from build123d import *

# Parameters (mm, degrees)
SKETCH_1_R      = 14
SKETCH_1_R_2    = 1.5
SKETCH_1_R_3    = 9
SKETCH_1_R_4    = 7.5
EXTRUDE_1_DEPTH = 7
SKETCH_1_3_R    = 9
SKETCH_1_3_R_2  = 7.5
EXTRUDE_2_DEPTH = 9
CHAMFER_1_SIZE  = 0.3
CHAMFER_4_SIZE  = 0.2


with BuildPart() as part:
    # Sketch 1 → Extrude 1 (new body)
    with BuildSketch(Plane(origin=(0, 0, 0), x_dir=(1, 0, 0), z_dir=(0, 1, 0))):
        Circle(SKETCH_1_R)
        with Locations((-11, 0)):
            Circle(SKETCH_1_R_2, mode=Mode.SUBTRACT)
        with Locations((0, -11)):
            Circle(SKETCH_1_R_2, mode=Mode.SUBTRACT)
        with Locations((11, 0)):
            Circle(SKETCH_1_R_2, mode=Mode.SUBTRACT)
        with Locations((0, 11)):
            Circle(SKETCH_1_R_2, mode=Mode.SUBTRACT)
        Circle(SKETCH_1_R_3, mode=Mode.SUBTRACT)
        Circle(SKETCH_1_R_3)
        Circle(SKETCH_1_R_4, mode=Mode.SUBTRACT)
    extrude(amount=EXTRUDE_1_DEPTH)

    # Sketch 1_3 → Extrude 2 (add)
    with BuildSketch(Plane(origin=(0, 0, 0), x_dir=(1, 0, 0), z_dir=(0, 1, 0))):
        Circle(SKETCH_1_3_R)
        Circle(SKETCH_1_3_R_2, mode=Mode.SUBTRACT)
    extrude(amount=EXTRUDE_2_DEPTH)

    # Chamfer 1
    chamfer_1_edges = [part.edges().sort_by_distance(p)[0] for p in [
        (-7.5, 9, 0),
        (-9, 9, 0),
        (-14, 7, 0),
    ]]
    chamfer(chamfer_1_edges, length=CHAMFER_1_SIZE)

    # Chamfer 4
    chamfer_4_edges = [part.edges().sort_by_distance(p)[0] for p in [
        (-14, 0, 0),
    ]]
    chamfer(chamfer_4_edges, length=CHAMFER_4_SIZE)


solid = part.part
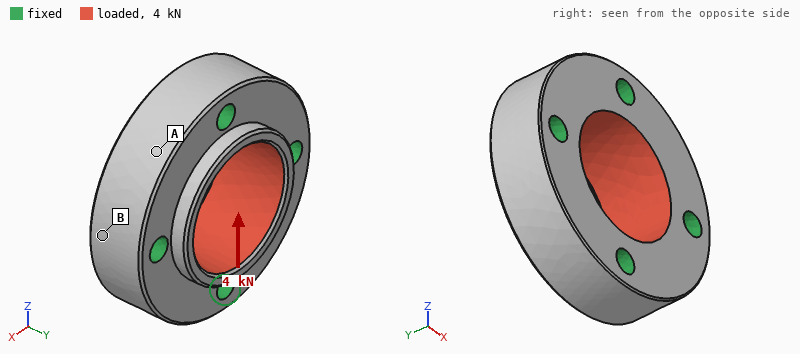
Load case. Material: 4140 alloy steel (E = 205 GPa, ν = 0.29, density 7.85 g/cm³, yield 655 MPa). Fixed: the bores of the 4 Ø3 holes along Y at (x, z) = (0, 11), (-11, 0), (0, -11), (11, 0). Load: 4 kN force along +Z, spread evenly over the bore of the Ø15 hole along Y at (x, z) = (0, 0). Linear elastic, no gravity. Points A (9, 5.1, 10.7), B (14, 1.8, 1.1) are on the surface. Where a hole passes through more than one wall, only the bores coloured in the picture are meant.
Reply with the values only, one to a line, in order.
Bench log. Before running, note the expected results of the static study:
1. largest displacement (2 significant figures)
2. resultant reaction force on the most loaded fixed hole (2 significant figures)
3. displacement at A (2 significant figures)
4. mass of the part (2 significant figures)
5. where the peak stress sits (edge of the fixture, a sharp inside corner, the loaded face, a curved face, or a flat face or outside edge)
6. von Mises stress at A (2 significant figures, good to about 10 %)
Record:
1.4 µm
1.1 kN
0.59 µm
24 g
edge of the fixture
12 MPa
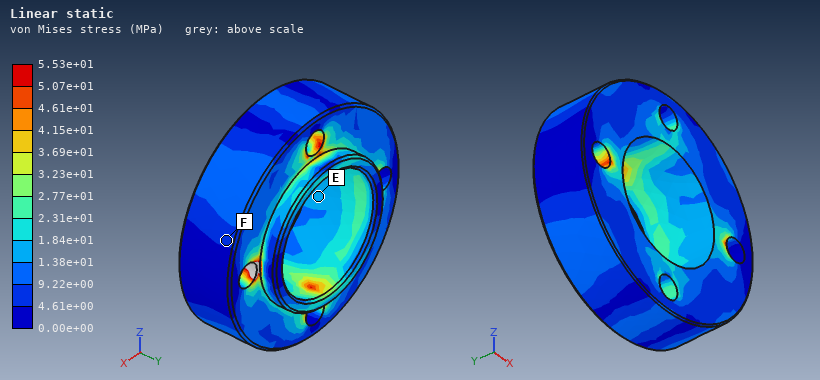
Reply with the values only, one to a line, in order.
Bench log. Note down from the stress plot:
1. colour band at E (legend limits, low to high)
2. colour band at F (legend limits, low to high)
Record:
1.38e+01 to 1.84e+01 MPa
4.61e+00 to 9.22e+00 MPa
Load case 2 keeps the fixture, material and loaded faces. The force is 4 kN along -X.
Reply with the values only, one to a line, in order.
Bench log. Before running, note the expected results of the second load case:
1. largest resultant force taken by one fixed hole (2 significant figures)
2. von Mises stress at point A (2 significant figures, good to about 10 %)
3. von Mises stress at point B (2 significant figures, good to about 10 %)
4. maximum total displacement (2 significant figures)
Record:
1.1 kN
11 MPa
9.5 MPa
1.4 µm
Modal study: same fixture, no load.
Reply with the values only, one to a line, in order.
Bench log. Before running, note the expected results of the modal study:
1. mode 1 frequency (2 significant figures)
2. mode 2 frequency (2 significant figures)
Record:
70 kHz
73 kHz
